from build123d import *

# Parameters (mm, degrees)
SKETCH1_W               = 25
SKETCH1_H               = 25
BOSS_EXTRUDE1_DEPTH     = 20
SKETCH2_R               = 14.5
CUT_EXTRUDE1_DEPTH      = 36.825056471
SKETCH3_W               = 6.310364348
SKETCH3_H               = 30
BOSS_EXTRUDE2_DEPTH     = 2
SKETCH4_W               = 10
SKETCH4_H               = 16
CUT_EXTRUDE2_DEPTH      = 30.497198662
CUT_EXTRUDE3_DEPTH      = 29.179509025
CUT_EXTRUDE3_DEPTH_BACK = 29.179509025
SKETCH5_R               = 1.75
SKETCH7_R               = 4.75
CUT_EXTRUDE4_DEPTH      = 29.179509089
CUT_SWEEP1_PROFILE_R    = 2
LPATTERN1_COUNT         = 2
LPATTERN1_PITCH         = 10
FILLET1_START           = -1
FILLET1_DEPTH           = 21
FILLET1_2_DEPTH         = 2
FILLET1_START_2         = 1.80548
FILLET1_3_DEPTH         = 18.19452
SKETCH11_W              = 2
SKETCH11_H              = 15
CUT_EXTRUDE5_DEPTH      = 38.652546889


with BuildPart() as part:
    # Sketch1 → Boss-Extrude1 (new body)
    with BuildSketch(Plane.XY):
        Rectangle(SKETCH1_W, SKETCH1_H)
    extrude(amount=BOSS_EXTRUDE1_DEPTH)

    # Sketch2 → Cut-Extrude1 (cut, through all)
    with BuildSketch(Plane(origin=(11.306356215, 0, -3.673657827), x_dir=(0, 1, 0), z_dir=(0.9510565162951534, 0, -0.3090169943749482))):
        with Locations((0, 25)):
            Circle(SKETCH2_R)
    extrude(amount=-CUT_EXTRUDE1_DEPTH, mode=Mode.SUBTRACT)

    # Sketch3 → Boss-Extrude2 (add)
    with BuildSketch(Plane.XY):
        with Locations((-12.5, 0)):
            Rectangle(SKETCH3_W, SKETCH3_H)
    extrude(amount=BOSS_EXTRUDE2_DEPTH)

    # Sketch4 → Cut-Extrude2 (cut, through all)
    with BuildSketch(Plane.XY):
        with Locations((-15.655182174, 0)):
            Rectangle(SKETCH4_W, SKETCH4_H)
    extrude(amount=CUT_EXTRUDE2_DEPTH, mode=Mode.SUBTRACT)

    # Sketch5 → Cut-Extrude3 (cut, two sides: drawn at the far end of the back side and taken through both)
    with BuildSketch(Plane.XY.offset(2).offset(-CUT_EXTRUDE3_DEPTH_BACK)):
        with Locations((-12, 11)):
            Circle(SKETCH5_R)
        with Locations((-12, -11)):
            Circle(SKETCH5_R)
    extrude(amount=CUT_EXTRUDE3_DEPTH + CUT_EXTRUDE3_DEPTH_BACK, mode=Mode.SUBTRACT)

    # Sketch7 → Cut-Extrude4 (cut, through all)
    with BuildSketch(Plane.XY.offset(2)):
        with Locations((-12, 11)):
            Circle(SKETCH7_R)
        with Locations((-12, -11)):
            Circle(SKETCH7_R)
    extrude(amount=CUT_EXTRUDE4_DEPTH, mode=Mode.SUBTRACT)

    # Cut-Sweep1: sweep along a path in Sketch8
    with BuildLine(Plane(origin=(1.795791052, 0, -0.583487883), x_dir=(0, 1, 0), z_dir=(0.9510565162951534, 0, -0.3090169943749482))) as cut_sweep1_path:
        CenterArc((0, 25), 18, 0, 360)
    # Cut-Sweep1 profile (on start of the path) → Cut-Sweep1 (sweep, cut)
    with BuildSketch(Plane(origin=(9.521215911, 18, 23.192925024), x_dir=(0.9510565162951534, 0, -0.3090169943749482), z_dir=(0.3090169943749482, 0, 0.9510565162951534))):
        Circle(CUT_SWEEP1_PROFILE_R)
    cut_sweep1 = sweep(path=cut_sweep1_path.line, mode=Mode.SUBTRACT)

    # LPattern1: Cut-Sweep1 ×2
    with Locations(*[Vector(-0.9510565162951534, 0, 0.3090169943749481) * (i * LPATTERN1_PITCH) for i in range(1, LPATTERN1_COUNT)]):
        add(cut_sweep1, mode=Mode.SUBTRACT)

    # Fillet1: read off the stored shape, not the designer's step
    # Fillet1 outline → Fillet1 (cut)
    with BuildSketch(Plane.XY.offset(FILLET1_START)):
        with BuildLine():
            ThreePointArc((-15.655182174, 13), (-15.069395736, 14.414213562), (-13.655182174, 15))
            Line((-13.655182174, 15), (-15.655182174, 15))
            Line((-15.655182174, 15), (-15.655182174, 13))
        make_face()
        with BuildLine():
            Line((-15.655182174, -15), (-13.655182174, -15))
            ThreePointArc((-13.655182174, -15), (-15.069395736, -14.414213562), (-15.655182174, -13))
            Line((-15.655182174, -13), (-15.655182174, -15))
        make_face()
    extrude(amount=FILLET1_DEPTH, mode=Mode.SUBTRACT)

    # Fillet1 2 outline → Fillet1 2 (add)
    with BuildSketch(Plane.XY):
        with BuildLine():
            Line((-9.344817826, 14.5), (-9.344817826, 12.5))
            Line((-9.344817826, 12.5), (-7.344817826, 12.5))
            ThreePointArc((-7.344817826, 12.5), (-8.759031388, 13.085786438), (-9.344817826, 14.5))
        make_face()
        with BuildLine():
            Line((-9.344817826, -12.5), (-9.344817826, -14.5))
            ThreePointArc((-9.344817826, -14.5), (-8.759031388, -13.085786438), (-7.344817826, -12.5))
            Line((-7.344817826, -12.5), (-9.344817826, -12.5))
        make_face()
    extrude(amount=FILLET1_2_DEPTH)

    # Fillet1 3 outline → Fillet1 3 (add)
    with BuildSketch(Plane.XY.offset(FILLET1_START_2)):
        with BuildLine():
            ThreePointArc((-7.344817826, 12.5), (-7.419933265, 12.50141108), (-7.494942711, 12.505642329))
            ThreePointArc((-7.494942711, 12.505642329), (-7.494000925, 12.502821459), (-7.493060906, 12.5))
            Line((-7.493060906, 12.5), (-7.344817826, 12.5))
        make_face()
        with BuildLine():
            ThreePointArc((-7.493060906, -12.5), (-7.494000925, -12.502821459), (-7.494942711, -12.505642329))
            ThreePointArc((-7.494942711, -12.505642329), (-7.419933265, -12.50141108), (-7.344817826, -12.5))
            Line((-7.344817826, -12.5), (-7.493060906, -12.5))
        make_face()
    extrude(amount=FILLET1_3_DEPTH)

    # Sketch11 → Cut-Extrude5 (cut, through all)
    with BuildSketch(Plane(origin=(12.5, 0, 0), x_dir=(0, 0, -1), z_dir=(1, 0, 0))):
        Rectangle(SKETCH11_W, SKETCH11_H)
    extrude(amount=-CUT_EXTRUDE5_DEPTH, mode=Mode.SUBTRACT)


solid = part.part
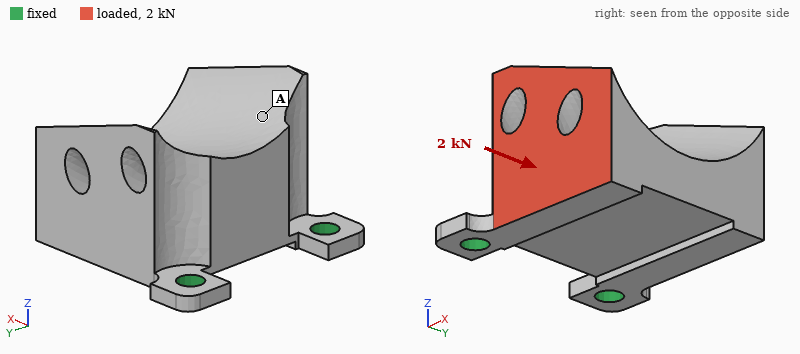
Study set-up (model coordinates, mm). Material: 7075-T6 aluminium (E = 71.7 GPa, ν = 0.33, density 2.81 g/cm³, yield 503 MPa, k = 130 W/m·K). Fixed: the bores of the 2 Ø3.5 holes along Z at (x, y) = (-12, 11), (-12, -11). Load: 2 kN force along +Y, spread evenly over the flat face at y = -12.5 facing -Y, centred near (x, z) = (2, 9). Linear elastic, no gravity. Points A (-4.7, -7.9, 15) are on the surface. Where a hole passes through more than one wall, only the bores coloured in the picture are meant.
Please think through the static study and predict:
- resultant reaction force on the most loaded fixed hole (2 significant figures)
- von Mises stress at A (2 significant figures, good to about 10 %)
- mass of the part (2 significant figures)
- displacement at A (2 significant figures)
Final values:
1.7 kN
36 MPa
17 g
47 µm
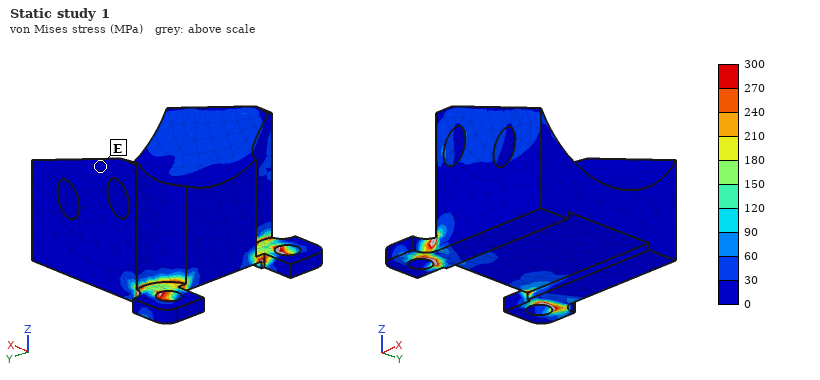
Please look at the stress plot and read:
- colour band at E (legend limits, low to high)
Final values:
0 to 30 MPa
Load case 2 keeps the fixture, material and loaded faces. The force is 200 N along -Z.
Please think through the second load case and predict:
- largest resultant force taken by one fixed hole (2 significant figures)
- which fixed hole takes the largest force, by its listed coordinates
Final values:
240 N
(-12, -11)
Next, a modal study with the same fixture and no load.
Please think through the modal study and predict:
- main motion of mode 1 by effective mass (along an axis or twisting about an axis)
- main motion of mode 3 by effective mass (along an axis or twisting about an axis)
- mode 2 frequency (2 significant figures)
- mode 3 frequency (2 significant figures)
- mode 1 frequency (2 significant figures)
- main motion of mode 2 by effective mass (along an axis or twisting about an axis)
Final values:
along Z
along Y
8900 Hz
12 kHz
1200 Hz
along Y
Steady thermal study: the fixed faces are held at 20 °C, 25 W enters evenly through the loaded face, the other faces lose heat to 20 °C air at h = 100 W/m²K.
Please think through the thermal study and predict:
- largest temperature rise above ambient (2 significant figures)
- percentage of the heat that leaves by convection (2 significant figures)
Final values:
42 K
33 %
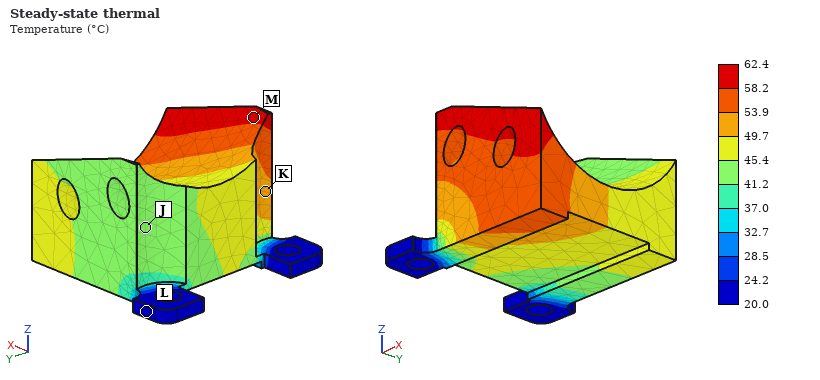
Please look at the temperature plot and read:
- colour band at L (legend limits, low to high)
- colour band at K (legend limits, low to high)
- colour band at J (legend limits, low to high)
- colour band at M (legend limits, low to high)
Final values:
20.0 to 24.2 °C
49.7 to 53.9 °C
41.2 to 45.4 °C
58.2 to 62.4 °C
